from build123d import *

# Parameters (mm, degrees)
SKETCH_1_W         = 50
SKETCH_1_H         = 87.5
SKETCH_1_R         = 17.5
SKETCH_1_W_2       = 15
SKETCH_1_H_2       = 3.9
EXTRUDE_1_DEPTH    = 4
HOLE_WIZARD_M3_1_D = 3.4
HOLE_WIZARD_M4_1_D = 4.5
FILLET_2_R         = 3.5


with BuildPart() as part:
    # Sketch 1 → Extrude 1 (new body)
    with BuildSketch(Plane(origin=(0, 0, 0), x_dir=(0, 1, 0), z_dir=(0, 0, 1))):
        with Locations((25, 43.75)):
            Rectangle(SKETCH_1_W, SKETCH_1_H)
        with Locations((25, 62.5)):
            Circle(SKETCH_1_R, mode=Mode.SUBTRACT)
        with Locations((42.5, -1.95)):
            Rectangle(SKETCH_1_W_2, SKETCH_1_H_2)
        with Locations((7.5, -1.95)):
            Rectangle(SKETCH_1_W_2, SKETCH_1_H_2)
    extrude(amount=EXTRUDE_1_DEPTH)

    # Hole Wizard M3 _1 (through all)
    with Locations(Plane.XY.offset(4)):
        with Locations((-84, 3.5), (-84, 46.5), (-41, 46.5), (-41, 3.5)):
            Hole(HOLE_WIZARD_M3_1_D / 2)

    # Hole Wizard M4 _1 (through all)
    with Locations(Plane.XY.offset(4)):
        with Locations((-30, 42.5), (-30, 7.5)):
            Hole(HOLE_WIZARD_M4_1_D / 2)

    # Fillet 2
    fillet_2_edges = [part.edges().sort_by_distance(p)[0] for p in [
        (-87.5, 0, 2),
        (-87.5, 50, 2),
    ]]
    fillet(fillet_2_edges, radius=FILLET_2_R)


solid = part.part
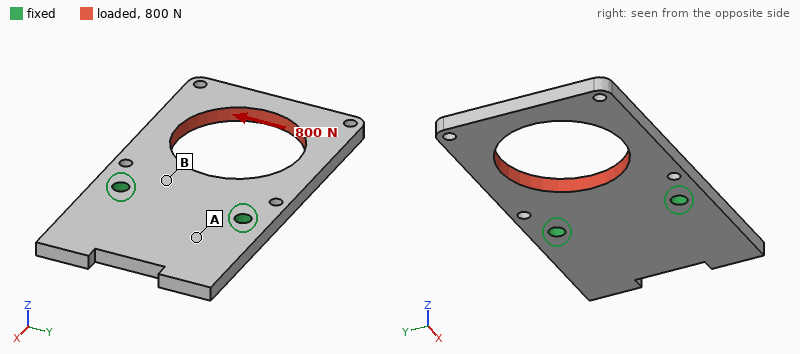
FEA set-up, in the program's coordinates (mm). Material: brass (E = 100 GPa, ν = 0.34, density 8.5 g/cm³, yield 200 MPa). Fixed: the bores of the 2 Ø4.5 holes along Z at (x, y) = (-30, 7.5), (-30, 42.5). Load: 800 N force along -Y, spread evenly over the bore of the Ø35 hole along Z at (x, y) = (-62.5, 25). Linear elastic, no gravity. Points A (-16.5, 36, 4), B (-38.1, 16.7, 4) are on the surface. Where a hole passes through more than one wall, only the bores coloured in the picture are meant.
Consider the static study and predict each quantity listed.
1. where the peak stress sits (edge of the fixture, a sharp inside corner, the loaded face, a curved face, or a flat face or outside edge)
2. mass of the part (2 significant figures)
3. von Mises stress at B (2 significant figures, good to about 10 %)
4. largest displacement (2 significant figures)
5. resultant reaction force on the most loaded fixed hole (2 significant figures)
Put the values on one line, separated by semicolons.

a curved face; 120 g; 15 MPa; 43 µm; 790 N
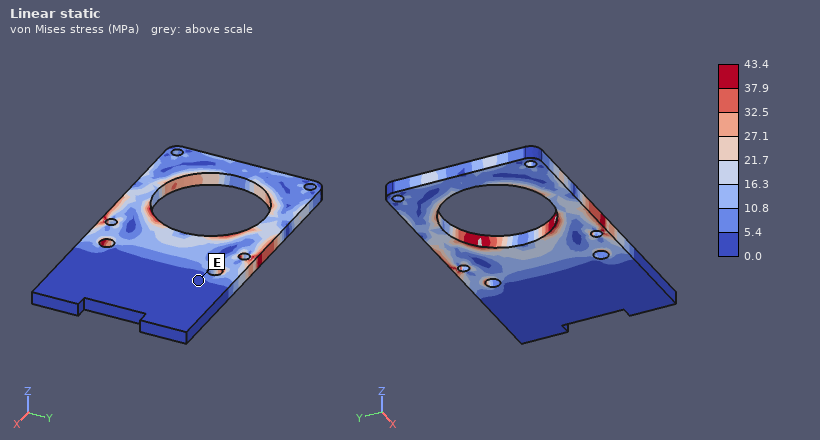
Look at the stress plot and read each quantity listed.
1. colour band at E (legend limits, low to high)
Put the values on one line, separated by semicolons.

0.0 to 5.4 MPa
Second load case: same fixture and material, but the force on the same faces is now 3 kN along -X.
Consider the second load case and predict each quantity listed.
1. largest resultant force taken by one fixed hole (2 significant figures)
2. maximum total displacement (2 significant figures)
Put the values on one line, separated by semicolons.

1.5 kN; 32 µm
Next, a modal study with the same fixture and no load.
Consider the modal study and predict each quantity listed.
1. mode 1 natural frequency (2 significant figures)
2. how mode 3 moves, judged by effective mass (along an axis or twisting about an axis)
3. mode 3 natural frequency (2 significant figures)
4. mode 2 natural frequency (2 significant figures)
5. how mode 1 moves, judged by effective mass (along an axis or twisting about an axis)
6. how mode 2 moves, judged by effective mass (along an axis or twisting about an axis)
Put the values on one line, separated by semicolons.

630 Hz; along Z; 2000 Hz; 1500 Hz; along Z; twisting about X
